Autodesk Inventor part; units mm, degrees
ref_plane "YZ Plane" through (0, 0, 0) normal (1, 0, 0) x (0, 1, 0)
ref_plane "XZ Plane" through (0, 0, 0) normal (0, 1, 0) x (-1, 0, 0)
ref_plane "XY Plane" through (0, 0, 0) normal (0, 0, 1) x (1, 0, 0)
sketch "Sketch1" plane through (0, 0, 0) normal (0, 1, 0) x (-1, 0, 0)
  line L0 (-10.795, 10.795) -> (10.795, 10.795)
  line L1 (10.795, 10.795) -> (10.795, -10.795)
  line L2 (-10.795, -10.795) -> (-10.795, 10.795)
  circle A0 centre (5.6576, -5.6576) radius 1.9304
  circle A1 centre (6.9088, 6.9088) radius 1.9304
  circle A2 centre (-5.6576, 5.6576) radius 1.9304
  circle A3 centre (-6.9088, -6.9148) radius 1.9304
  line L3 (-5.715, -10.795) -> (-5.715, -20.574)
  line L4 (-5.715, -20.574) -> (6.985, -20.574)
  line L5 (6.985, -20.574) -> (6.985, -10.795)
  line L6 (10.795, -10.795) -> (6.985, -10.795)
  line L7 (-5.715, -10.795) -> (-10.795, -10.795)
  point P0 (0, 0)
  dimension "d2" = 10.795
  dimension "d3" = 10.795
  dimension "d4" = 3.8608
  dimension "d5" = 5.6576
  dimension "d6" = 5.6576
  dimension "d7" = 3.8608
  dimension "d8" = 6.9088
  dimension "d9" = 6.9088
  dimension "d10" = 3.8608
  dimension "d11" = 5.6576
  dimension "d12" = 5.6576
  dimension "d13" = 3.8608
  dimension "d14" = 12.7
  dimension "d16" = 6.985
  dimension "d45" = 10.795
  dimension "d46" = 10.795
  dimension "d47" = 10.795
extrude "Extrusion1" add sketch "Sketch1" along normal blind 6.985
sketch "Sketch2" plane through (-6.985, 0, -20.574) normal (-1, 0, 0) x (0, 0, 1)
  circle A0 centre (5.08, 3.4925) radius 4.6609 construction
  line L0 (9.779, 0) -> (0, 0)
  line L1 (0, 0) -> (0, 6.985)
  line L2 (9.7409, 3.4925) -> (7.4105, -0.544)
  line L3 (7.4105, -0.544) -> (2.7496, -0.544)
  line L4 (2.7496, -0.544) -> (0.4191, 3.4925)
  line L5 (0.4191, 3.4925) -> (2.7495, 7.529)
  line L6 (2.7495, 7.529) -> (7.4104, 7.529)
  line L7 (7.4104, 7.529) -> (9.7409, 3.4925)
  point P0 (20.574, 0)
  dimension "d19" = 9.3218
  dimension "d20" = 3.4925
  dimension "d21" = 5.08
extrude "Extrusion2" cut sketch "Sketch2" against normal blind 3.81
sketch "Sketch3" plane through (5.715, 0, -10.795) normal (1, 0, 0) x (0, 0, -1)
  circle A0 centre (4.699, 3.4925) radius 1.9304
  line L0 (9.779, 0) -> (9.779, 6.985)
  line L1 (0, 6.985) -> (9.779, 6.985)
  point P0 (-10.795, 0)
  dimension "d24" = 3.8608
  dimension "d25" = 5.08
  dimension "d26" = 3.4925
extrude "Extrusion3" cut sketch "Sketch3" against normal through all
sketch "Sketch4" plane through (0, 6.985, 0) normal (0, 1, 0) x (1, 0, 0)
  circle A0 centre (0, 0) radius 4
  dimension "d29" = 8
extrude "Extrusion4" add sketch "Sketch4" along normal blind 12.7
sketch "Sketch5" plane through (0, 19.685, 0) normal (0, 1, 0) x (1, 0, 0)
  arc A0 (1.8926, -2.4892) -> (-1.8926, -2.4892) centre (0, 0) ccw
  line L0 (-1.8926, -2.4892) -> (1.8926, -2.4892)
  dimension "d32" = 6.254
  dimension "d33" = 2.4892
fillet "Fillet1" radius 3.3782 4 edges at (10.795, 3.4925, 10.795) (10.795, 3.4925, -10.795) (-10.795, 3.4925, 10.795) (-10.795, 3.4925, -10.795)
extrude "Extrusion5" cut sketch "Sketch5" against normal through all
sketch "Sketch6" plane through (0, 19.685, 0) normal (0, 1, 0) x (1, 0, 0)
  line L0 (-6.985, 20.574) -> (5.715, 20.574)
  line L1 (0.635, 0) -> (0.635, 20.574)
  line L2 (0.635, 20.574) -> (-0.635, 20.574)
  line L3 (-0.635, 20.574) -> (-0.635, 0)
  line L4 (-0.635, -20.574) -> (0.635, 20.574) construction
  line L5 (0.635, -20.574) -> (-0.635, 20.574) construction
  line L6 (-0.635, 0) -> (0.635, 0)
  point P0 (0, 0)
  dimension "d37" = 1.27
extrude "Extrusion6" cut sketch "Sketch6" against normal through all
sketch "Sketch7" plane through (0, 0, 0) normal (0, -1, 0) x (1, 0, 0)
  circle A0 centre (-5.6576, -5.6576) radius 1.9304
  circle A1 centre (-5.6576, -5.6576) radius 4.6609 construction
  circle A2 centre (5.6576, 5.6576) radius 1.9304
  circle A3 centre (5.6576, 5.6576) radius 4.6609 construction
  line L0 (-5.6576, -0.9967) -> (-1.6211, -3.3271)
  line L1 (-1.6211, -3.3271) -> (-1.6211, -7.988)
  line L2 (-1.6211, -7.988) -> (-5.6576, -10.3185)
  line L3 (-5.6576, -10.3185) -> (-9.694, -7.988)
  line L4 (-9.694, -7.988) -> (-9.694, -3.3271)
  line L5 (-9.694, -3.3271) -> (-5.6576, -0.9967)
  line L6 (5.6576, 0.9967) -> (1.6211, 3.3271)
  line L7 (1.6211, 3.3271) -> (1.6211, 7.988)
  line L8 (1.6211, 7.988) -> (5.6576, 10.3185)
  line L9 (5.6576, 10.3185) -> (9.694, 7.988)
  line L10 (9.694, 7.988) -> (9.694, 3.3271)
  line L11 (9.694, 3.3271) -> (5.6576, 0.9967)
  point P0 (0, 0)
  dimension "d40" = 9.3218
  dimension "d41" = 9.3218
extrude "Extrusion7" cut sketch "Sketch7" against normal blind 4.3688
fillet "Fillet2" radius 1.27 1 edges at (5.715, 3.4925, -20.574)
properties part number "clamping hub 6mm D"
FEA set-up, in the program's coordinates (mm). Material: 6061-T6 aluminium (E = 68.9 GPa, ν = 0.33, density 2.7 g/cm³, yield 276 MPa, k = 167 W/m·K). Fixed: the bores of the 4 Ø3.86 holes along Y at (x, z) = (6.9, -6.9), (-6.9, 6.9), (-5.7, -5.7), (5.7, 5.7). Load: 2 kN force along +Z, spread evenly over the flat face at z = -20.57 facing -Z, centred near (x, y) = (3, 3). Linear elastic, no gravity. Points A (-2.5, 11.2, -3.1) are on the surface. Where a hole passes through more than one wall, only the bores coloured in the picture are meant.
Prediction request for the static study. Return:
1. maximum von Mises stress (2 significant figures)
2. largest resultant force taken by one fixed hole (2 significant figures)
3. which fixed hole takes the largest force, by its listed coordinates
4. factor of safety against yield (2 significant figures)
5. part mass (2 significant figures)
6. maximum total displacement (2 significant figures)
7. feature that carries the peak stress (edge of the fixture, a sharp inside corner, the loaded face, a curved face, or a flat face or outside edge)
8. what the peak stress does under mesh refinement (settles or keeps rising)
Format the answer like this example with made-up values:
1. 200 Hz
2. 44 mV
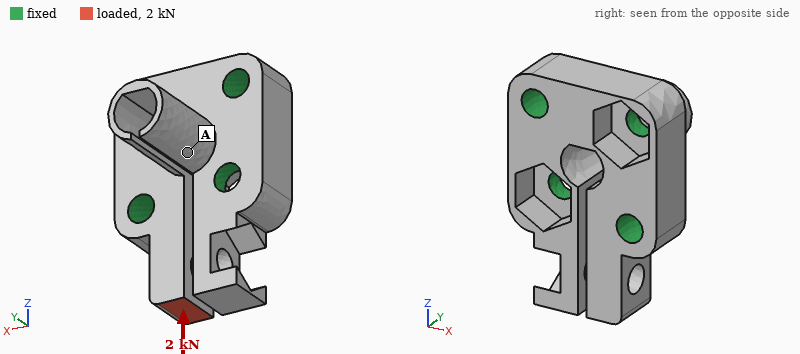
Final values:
1. 360 MPa
2. 1.9 kN
3. (6.9, -6.9)
4. 0.77
5. 8.0 g
6. 58 µm
7. a curved face
8. settles
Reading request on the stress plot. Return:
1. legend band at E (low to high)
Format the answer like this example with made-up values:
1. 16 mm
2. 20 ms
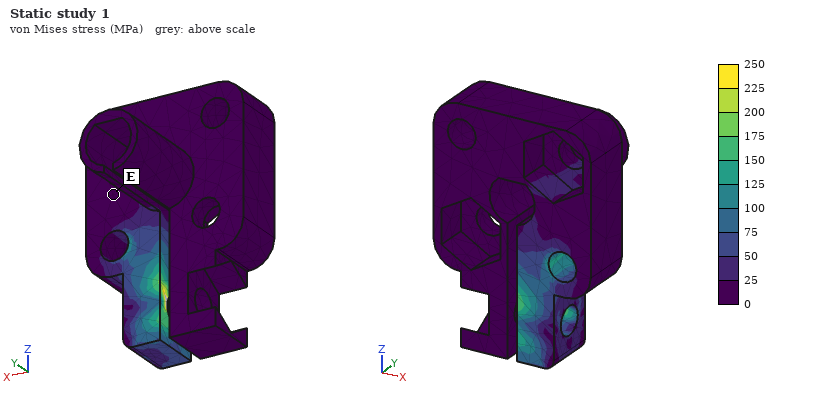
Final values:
1. 0 to 25 MPa
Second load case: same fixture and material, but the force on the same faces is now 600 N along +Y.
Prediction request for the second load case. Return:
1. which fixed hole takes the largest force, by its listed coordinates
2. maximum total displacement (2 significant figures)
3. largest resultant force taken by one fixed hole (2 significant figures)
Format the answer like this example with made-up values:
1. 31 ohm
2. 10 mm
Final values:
1. (6.9, -6.9)
2. 79 µm
3. 680 N
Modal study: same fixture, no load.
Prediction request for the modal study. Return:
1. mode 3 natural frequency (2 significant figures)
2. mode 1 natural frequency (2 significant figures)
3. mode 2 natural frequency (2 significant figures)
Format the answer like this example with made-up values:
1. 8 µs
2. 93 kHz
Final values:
1. 15 kHz
2. 12 kHz
3. 14 kHz
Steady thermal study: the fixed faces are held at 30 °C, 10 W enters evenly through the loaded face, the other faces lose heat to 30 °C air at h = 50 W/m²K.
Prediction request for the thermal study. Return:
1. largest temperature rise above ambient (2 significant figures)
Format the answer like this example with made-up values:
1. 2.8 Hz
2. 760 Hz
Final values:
1. 30 K
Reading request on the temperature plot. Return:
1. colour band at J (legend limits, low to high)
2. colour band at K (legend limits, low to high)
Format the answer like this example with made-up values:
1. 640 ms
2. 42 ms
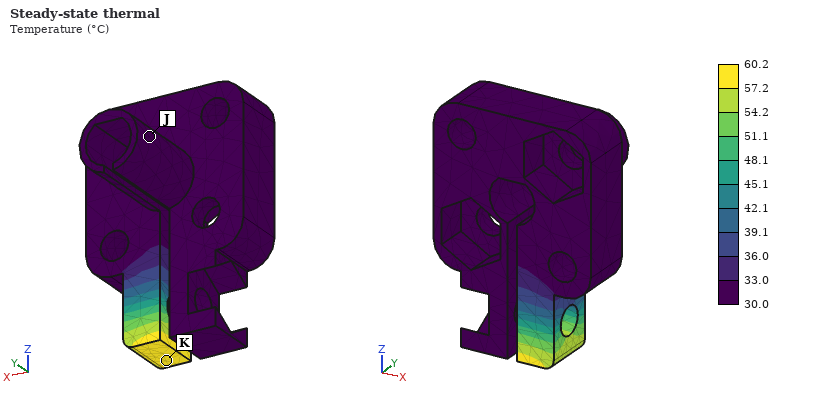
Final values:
1. 30.0 to 33.0 °C
2. 57.2 to 60.2 °C
